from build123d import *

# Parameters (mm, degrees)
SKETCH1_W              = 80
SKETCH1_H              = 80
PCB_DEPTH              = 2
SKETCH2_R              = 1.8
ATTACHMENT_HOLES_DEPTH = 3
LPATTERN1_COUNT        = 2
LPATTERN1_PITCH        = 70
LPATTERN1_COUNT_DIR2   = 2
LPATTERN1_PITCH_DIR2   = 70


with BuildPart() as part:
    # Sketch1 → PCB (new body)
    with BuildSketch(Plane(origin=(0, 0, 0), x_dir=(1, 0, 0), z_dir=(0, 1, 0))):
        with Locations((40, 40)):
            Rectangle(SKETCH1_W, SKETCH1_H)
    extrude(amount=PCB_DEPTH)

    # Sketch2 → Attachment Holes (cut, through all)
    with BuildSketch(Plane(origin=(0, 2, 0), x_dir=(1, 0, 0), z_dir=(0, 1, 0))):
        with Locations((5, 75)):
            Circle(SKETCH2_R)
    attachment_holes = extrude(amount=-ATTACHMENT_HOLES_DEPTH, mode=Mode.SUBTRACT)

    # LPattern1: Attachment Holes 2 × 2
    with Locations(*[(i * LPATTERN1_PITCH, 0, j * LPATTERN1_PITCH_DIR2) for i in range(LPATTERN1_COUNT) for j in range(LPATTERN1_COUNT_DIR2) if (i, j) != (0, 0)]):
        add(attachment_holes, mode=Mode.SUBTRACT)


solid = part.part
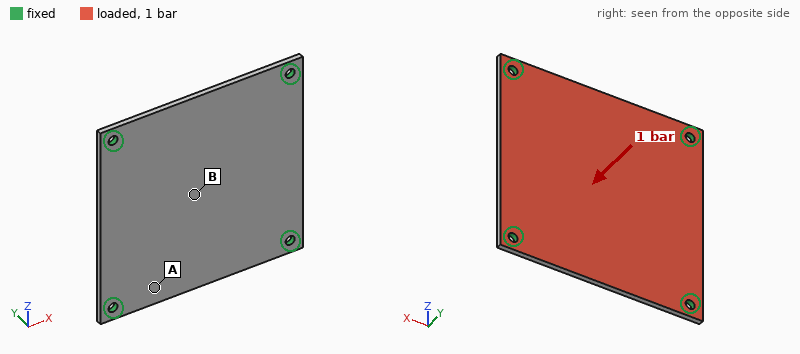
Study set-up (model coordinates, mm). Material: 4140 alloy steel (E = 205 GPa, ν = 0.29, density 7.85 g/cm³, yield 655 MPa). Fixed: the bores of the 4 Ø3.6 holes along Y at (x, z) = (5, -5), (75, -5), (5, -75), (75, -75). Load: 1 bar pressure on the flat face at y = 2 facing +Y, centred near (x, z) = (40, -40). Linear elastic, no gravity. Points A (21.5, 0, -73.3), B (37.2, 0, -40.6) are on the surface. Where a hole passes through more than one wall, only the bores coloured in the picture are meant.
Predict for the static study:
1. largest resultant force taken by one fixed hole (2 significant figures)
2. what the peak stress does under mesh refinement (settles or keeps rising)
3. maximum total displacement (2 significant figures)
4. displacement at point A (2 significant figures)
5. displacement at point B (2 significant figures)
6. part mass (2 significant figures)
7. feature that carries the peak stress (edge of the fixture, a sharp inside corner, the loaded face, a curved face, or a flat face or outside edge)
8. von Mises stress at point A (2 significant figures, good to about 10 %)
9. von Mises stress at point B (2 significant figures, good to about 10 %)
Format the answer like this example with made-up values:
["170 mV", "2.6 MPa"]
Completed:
["160 N", "keeps rising", "0.13 mm", "0.040 mm", "0.13 mm", "100 g", "edge of the fixture", "16 MPa", "40 MPa"]
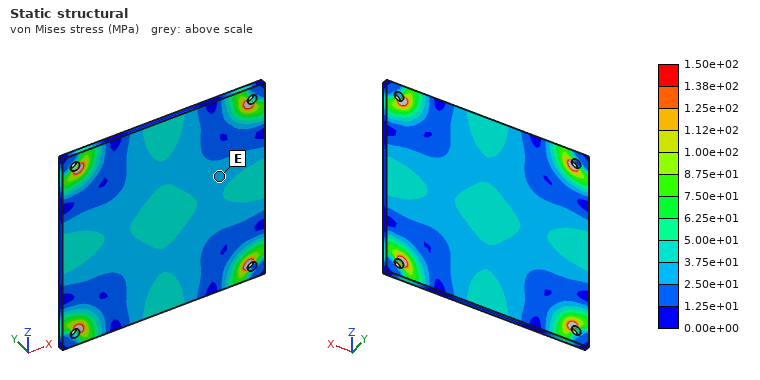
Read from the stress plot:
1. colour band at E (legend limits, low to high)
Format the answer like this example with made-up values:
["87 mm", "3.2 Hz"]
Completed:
["2.50e+01 to 3.75e+01 MPa"]
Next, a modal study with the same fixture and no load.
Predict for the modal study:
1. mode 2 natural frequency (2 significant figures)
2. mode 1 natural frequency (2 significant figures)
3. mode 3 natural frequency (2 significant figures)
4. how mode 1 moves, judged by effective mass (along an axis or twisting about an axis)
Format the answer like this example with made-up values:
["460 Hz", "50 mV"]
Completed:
["2400 Hz", "1400 Hz", "2400 Hz", "along Y"]
